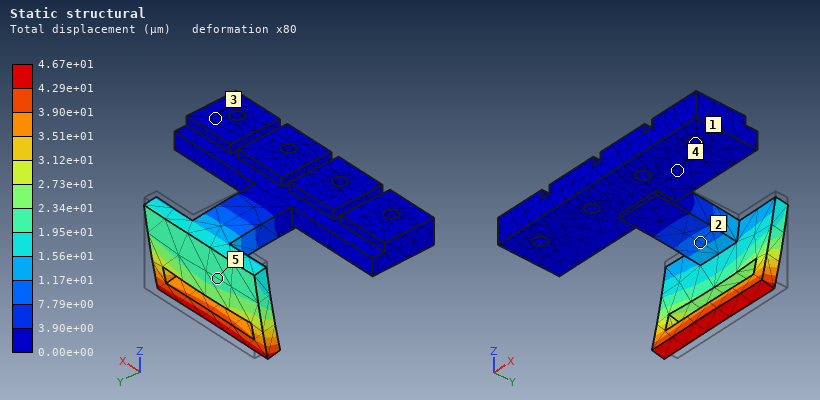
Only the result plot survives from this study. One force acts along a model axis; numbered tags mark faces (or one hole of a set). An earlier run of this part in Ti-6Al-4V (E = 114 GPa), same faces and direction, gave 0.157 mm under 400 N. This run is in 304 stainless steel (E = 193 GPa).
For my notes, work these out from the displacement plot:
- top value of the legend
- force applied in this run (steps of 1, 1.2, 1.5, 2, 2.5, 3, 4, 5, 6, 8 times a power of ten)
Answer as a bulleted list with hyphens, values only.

- 4.67e+01 µm
- 200 N
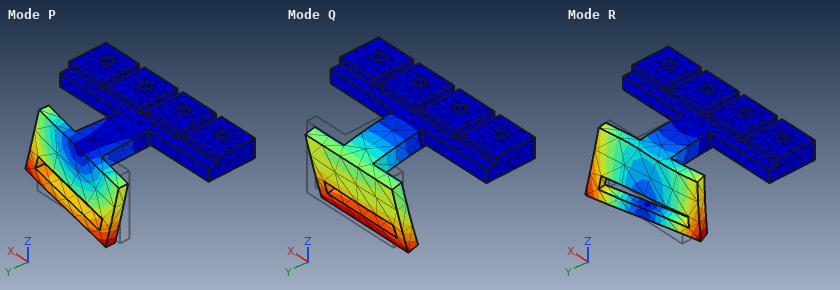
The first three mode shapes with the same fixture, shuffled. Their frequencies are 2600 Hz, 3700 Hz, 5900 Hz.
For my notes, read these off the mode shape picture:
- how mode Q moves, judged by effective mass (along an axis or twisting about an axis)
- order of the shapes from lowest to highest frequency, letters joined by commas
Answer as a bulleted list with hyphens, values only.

- along Z
- Q, P, R
